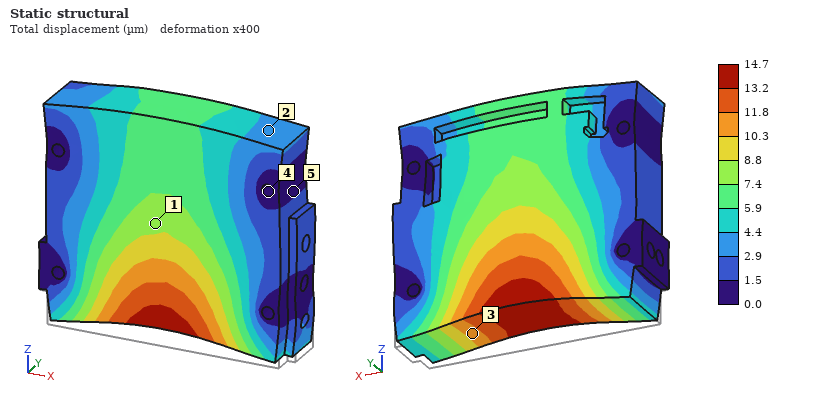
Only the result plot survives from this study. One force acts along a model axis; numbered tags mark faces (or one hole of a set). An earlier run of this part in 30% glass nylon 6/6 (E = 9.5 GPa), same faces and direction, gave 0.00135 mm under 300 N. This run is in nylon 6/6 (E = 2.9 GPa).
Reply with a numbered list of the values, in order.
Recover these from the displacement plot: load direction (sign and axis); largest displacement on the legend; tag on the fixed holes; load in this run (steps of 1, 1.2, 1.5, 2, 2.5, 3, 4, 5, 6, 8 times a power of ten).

1. +Z
2. 14.7 µm
3. 4
4. 1 kN
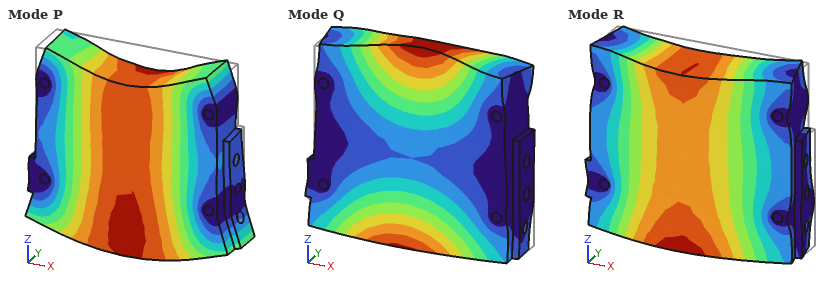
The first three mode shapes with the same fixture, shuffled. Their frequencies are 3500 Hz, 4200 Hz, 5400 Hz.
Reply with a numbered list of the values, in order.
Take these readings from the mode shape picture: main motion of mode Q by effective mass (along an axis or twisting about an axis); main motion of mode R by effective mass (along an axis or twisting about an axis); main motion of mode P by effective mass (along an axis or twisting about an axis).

1. twisting about X
2. along Y
3. along Z
